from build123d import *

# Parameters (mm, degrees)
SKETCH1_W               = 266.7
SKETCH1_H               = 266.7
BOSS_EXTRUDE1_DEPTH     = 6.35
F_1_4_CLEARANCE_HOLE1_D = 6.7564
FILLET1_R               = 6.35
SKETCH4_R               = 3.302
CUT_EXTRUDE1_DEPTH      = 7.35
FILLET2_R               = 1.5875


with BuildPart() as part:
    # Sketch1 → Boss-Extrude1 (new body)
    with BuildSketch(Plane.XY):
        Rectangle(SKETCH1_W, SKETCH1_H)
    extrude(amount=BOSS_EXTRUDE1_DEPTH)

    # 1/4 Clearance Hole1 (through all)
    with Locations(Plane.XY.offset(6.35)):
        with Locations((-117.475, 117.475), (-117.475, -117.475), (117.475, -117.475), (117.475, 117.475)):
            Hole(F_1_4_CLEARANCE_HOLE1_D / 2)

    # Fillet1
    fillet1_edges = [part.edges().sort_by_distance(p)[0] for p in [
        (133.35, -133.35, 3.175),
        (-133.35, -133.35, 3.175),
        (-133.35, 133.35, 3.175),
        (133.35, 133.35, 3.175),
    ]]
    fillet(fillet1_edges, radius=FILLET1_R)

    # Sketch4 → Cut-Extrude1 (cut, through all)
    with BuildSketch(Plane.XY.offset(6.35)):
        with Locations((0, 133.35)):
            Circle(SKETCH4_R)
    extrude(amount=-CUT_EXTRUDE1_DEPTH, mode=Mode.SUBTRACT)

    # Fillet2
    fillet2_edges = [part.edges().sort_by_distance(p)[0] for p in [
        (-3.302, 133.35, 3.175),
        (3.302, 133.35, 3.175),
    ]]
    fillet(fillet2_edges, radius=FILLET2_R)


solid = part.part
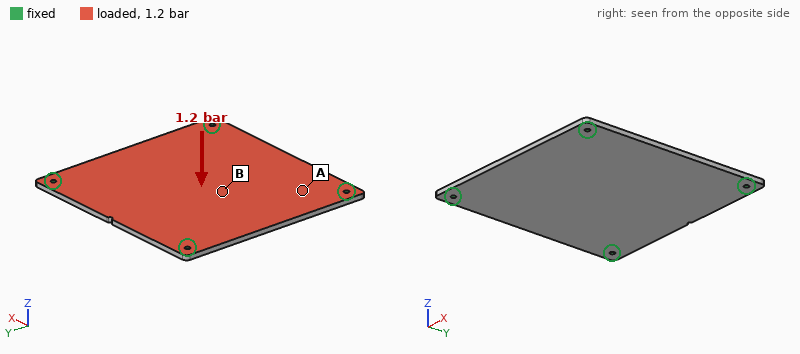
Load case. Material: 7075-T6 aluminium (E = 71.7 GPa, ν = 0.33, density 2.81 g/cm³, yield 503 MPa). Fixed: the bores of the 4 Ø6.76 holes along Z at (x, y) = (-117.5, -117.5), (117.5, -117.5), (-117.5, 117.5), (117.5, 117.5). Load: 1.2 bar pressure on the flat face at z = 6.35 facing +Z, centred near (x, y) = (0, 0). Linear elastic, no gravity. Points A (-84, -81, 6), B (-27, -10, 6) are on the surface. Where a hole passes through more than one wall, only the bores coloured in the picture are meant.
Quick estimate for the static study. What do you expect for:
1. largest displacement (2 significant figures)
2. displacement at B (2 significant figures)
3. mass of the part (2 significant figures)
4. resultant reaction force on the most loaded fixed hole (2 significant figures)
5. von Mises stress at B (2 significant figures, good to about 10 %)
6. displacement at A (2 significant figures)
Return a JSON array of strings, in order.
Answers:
["1.9 mm", "1.8 mm", "1.3 kg", "2.1 kN", "57 MPa", "0.73 mm"]
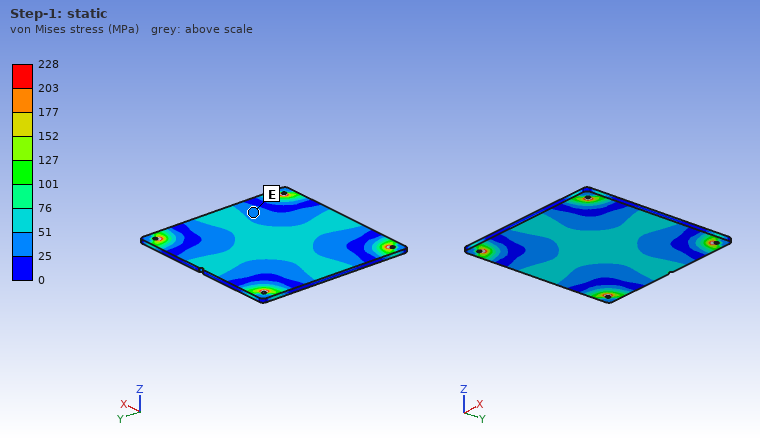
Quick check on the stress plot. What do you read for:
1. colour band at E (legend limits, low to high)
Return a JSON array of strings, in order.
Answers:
["25 to 51 MPa"]
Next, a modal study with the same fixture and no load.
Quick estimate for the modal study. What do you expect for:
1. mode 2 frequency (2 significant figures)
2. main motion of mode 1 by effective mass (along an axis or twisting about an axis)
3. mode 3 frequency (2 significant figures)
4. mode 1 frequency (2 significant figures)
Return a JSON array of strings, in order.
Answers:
["640 Hz", "along Z", "640 Hz", "360 Hz"]
